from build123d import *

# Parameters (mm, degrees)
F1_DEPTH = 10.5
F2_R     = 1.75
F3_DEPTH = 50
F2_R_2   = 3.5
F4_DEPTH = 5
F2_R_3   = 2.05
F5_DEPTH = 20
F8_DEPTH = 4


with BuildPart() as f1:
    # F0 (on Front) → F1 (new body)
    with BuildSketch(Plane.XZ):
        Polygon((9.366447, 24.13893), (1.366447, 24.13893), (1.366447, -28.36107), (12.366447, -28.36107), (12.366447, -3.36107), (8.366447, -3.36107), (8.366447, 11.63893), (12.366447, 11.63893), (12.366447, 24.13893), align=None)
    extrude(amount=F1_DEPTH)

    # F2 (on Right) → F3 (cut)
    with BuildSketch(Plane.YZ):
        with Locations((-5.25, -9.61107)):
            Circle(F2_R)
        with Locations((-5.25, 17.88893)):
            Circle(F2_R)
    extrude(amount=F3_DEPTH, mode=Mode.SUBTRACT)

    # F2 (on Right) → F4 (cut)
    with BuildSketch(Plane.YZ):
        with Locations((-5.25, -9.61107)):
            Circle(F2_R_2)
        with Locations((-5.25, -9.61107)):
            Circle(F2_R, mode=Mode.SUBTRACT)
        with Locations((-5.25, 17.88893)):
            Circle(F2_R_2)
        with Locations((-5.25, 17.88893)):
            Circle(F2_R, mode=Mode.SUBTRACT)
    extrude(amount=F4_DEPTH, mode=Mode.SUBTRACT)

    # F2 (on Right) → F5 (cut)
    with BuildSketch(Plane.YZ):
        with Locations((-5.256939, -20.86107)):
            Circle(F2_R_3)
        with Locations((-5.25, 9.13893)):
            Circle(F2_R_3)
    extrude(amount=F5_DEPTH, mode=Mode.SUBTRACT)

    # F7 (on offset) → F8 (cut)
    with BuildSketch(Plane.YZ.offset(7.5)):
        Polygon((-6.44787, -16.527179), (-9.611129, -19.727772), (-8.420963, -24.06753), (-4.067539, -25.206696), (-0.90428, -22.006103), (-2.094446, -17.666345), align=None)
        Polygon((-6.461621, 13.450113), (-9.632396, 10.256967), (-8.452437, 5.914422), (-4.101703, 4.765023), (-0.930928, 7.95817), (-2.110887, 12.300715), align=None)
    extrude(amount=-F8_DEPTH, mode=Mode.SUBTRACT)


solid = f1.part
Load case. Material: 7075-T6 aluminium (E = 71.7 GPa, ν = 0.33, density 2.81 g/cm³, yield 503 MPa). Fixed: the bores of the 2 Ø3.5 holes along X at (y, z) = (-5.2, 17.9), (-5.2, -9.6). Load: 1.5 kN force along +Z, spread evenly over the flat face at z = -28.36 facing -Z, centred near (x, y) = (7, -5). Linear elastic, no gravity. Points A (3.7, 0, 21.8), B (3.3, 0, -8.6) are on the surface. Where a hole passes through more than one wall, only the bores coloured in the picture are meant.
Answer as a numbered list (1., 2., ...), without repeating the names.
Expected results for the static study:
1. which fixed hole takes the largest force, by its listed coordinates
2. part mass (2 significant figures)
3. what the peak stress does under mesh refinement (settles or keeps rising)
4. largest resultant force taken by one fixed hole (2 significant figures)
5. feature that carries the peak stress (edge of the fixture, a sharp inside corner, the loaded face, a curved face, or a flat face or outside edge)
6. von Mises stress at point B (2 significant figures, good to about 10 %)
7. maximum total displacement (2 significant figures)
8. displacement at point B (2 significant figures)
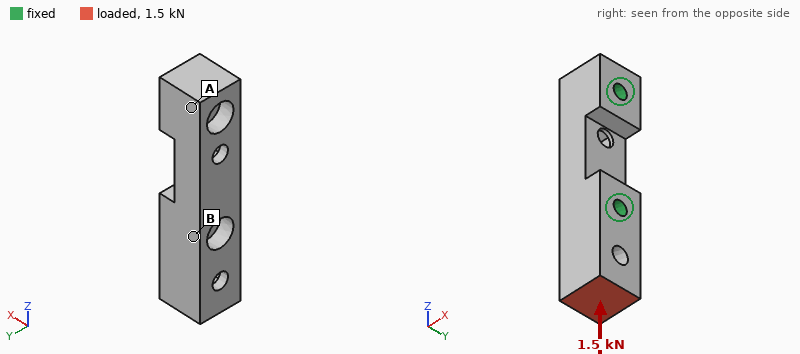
1. (-5.2, -9.6)
2. 13 g
3. keeps rising
4. 1.4 kN
5. edge of the fixture
6. 11 MPa
7. 10 µm
8. 1.7 µm
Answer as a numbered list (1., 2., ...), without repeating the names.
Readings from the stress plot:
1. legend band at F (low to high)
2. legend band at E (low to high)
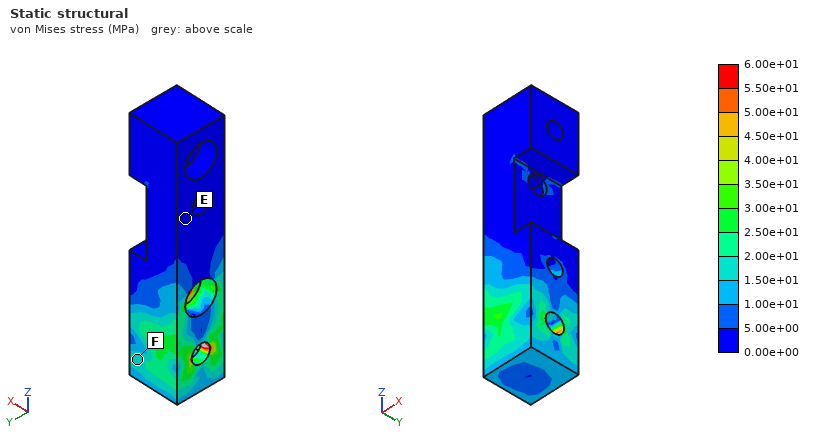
1. 1.50e+01 to 2.00e+01 MPa
2. 0.00e+00 to 5.00e+00 MPa
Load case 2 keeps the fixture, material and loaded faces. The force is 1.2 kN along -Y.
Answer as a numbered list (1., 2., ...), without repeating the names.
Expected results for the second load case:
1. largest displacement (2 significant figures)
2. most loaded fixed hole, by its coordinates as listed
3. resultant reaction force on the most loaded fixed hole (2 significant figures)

1. 89 µm
2. (-5.2, -9.6)
3. 1.5 kN
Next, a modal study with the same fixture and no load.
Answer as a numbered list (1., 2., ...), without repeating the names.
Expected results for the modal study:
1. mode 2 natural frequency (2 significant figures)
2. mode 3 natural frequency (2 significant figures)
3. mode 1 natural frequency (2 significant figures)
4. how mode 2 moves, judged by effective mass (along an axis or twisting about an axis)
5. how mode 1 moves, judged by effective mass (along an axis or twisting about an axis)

1. 16 kHz
2. 31 kHz
3. 15 kHz
4. along X
5. along Y
